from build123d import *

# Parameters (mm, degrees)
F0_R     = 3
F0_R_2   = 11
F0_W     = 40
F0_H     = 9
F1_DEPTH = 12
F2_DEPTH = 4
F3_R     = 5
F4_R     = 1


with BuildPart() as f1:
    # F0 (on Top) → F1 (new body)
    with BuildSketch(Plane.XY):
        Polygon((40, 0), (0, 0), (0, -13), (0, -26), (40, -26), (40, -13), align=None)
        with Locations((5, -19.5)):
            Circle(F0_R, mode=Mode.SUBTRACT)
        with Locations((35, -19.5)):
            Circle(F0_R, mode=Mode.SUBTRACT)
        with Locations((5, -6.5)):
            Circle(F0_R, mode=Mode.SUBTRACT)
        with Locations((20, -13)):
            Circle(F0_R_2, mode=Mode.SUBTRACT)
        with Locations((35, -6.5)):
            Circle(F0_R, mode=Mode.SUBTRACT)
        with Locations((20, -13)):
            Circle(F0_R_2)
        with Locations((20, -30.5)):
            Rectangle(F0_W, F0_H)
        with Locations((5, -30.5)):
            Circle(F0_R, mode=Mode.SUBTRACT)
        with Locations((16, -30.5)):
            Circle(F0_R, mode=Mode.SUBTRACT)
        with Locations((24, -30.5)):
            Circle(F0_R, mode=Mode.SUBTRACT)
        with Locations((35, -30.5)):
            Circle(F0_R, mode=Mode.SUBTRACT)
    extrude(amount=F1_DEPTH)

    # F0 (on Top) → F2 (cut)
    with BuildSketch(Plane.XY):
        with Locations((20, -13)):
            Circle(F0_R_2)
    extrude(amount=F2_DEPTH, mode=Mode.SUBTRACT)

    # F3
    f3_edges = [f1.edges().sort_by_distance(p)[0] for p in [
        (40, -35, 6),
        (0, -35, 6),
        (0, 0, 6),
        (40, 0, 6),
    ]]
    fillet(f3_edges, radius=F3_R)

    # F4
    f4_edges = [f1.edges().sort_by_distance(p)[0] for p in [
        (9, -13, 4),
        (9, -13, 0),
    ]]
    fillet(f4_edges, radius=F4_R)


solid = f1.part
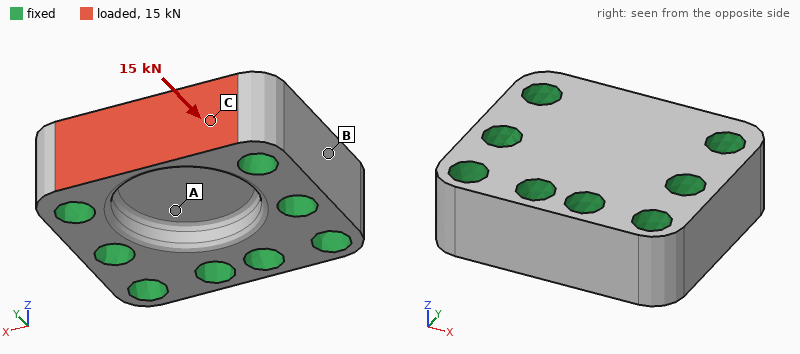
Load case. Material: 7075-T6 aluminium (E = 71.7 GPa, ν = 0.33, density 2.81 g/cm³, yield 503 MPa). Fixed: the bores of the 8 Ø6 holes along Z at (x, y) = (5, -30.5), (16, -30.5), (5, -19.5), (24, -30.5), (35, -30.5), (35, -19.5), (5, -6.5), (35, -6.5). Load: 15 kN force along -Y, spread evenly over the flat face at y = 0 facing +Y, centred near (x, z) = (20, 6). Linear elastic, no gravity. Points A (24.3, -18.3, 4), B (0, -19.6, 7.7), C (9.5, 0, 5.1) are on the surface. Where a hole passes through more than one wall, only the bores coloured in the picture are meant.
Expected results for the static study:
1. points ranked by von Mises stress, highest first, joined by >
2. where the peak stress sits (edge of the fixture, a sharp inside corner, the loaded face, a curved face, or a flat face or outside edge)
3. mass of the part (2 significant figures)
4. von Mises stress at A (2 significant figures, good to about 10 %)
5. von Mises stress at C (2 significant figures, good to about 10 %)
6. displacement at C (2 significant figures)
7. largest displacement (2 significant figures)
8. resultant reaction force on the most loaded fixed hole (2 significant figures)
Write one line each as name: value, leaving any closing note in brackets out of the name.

points ranked by von Mises stress, highest first, joined by >: C > A > B
where the peak stress sits: a curved face
mass of the part: 35 g
von Mises stress at A: 26 MPa
von Mises stress at C: 60 MPa
displacement at C: 7.4 µm
largest displacement: 44 µm
resultant reaction force on the most loaded fixed hole: 5.0 kN
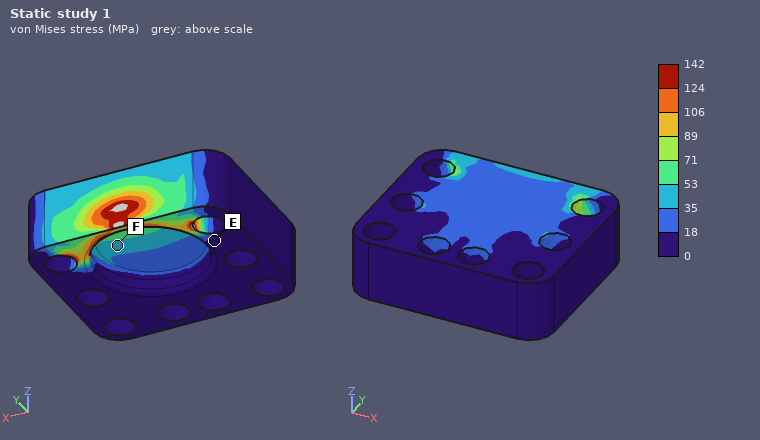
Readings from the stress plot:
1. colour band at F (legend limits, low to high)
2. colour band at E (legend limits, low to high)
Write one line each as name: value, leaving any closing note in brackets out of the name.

colour band at F: 35 to 53 MPa
colour band at E: 0 to 18 MPa
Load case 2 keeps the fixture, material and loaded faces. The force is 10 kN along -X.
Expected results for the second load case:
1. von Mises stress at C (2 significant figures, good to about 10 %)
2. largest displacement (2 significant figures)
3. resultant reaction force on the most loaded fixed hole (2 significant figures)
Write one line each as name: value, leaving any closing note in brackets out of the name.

von Mises stress at C: 58 MPa
largest displacement: 10 µm
resultant reaction force on the most loaded fixed hole: 4.9 kN
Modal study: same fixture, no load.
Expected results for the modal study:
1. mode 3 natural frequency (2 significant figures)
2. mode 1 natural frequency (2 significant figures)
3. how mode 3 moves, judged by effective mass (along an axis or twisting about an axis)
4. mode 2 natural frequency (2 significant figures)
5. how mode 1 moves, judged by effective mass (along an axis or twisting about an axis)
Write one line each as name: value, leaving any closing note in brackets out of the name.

mode 3 natural frequency: 71 kHz
mode 1 natural frequency: 49 kHz
how mode 3 moves, judged by effective mass: along Y
mode 2 natural frequency: 64 kHz
how mode 1 moves, judged by effective mass: along Z
